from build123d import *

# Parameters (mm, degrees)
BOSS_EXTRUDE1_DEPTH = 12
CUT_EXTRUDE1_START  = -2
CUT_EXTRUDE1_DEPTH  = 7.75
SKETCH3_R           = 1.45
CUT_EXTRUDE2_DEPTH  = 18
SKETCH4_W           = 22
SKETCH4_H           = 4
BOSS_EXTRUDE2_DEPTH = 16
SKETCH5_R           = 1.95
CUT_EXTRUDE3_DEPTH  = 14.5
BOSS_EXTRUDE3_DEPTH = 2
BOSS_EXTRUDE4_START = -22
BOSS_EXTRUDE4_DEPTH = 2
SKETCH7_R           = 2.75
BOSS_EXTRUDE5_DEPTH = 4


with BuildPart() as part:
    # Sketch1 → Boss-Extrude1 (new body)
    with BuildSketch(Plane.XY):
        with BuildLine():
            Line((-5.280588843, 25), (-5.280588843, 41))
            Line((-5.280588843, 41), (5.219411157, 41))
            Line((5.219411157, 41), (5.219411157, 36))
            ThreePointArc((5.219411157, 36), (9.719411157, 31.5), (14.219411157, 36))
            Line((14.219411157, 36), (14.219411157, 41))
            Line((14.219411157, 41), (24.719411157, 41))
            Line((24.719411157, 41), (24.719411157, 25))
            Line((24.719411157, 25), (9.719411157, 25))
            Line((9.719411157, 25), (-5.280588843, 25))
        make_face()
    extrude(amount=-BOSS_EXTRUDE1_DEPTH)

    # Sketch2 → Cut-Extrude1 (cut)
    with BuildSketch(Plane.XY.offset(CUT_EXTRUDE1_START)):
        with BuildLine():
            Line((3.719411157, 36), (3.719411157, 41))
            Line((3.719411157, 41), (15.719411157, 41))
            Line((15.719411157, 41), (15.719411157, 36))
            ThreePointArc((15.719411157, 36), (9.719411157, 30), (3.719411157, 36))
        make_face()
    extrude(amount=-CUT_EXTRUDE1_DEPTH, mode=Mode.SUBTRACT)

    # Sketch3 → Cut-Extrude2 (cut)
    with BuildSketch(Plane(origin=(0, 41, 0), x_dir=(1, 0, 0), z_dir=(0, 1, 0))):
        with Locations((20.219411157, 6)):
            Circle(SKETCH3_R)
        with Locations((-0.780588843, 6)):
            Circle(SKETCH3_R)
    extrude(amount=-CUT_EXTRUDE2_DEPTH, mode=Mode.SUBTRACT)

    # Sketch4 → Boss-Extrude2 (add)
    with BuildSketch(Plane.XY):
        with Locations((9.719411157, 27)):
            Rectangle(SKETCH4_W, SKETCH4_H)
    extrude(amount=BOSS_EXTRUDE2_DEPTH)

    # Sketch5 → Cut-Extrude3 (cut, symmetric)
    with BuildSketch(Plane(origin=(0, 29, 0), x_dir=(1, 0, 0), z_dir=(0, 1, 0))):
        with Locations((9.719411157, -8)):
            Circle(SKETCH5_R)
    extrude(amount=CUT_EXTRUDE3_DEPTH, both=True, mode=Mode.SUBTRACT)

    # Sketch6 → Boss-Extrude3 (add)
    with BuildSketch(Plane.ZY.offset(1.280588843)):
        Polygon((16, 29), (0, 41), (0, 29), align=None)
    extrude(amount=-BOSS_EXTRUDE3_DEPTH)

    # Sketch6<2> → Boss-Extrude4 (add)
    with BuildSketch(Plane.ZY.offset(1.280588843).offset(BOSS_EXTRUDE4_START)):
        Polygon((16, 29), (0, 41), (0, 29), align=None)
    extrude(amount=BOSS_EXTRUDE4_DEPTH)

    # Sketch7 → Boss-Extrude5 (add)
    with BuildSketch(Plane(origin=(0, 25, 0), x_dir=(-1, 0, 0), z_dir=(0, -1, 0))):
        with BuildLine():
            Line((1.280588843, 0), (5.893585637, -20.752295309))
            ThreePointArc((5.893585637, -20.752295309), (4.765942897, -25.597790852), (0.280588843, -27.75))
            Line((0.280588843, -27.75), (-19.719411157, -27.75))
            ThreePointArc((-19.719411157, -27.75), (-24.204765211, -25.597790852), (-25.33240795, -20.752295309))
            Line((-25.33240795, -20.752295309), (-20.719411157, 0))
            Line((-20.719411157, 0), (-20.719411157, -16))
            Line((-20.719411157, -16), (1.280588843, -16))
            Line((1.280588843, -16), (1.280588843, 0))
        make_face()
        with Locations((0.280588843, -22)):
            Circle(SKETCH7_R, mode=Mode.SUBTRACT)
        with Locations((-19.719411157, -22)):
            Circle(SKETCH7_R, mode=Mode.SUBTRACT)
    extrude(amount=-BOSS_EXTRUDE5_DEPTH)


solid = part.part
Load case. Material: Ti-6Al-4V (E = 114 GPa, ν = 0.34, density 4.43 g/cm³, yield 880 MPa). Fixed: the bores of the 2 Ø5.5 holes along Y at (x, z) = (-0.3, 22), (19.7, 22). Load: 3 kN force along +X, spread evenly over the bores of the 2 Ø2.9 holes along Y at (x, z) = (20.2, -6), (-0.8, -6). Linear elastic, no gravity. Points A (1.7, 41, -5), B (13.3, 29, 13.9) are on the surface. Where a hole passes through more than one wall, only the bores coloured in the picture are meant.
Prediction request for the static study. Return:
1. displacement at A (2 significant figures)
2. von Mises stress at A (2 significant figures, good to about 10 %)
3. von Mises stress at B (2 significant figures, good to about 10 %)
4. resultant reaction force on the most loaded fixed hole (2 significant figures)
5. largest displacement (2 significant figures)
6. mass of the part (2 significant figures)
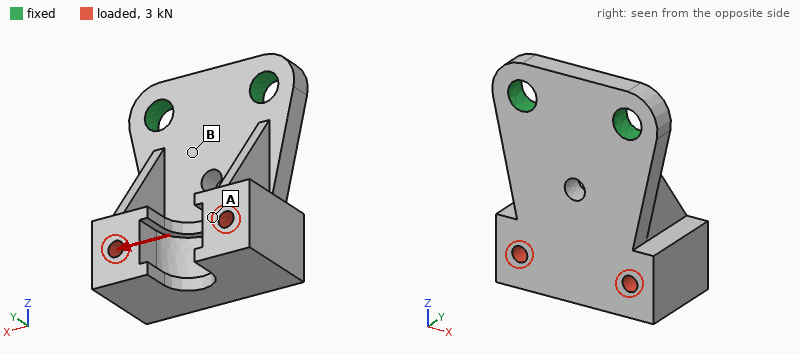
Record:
0.14 mm
29 MPa
120 MPa
4.0 kN
0.17 mm
33 g
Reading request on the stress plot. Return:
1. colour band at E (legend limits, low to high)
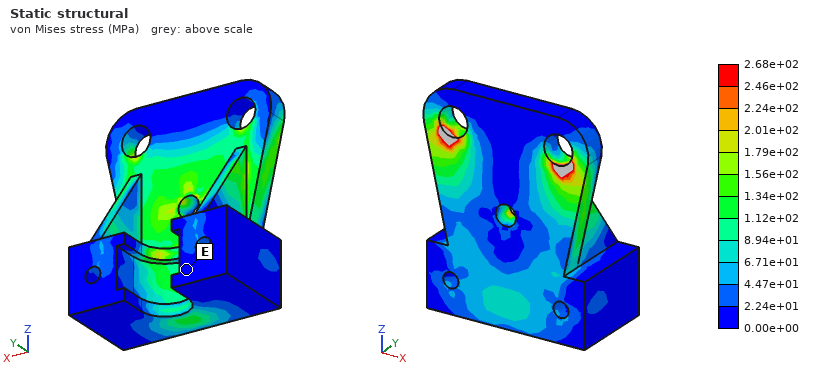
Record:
0.00e+00 to 2.24e+01 MPa
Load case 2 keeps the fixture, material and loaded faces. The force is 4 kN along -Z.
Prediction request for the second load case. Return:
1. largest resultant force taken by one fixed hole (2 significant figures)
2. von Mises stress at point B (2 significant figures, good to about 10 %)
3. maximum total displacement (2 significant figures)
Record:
2.0 kN
210 MPa
0.47 mm
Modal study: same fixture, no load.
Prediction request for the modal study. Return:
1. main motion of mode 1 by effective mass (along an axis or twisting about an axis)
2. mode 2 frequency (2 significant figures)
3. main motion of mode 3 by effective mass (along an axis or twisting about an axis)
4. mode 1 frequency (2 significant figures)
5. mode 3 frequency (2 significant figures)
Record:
along Y
4600 Hz
along X
1900 Hz
9600 Hz
